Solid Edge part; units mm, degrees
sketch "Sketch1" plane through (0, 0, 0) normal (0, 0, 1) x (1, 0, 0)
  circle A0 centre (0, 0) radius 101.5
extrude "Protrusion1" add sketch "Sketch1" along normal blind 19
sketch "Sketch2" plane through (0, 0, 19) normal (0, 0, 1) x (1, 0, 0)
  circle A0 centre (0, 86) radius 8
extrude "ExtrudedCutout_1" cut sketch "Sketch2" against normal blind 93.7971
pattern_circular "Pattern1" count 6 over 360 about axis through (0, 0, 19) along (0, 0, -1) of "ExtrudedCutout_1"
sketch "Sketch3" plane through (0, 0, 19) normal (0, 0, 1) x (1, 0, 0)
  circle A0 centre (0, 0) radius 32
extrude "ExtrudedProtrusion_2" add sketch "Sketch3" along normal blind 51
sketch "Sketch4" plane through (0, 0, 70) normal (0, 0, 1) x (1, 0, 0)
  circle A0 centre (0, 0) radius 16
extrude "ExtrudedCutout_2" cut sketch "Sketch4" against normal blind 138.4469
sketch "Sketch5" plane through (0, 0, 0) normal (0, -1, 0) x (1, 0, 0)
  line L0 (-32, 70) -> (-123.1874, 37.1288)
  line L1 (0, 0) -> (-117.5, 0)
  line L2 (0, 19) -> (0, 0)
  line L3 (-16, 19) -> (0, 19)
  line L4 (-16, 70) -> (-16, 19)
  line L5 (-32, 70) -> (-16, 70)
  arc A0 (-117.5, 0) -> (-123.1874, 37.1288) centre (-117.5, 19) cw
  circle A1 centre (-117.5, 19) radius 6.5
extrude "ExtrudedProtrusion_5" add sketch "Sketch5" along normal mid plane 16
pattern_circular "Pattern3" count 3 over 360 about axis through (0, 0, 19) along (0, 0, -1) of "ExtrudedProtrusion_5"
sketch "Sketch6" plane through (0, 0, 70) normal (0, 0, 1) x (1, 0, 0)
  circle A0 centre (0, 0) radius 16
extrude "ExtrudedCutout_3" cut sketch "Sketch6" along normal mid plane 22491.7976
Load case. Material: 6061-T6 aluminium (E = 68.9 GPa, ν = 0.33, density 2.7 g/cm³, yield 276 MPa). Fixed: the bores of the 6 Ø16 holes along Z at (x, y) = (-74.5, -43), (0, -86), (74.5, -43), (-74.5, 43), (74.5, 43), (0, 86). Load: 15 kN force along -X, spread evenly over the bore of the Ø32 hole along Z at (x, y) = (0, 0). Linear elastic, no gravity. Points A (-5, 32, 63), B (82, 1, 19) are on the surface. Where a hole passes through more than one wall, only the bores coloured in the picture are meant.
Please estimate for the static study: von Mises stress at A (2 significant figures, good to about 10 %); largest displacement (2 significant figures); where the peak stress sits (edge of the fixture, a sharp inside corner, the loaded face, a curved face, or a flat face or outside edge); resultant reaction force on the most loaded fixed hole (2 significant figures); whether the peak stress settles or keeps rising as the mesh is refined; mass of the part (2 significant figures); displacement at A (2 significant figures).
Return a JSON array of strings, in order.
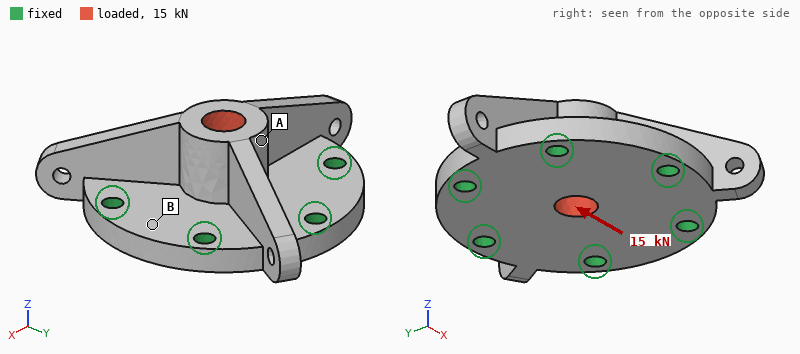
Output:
["3.3 MPa", "19 µm", "edge of the fixture", "3.9 kN", "keeps rising", "2.4 kg", "13 µm"]
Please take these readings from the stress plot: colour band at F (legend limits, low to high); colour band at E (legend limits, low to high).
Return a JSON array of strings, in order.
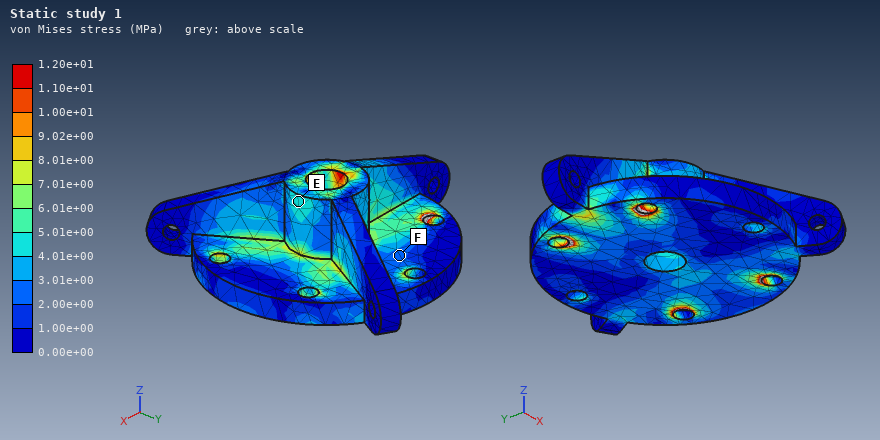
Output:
["2.00e+00 to 3.01e+00 MPa", "4.01e+00 to 5.01e+00 MPa"]
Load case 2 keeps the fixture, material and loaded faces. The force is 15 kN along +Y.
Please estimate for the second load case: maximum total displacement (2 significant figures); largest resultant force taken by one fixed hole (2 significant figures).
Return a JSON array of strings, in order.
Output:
["17 µm", "4.2 kN"]
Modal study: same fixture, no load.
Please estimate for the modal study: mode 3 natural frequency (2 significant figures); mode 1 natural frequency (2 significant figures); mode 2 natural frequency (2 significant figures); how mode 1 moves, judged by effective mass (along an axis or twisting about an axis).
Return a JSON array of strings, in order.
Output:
["5400 Hz", "5100 Hz", "5400 Hz", "along Z"]
